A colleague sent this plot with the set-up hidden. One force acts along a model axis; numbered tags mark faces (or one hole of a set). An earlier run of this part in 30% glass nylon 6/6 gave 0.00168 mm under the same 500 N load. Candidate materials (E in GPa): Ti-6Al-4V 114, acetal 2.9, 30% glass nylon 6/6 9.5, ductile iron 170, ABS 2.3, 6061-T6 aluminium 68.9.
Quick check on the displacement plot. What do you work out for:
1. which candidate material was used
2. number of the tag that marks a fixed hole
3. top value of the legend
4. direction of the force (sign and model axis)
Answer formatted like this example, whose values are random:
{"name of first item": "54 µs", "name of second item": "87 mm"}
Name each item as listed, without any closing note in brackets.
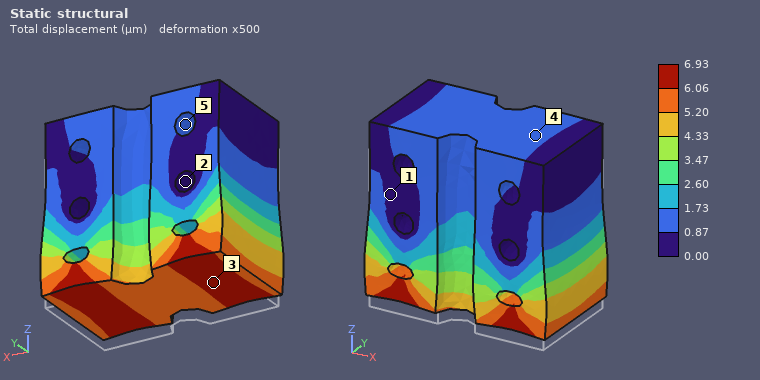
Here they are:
{"which candidate material was used": "ABS", "number of the tag that marks a fixed hole": "2", "top value of the legend": "6.93 µm", "direction of the force": "+Z"}
